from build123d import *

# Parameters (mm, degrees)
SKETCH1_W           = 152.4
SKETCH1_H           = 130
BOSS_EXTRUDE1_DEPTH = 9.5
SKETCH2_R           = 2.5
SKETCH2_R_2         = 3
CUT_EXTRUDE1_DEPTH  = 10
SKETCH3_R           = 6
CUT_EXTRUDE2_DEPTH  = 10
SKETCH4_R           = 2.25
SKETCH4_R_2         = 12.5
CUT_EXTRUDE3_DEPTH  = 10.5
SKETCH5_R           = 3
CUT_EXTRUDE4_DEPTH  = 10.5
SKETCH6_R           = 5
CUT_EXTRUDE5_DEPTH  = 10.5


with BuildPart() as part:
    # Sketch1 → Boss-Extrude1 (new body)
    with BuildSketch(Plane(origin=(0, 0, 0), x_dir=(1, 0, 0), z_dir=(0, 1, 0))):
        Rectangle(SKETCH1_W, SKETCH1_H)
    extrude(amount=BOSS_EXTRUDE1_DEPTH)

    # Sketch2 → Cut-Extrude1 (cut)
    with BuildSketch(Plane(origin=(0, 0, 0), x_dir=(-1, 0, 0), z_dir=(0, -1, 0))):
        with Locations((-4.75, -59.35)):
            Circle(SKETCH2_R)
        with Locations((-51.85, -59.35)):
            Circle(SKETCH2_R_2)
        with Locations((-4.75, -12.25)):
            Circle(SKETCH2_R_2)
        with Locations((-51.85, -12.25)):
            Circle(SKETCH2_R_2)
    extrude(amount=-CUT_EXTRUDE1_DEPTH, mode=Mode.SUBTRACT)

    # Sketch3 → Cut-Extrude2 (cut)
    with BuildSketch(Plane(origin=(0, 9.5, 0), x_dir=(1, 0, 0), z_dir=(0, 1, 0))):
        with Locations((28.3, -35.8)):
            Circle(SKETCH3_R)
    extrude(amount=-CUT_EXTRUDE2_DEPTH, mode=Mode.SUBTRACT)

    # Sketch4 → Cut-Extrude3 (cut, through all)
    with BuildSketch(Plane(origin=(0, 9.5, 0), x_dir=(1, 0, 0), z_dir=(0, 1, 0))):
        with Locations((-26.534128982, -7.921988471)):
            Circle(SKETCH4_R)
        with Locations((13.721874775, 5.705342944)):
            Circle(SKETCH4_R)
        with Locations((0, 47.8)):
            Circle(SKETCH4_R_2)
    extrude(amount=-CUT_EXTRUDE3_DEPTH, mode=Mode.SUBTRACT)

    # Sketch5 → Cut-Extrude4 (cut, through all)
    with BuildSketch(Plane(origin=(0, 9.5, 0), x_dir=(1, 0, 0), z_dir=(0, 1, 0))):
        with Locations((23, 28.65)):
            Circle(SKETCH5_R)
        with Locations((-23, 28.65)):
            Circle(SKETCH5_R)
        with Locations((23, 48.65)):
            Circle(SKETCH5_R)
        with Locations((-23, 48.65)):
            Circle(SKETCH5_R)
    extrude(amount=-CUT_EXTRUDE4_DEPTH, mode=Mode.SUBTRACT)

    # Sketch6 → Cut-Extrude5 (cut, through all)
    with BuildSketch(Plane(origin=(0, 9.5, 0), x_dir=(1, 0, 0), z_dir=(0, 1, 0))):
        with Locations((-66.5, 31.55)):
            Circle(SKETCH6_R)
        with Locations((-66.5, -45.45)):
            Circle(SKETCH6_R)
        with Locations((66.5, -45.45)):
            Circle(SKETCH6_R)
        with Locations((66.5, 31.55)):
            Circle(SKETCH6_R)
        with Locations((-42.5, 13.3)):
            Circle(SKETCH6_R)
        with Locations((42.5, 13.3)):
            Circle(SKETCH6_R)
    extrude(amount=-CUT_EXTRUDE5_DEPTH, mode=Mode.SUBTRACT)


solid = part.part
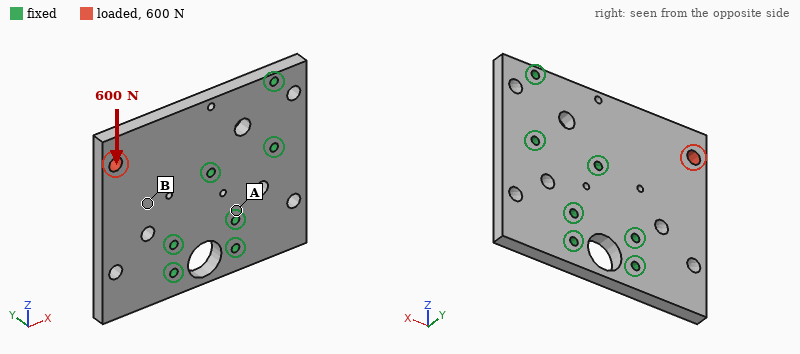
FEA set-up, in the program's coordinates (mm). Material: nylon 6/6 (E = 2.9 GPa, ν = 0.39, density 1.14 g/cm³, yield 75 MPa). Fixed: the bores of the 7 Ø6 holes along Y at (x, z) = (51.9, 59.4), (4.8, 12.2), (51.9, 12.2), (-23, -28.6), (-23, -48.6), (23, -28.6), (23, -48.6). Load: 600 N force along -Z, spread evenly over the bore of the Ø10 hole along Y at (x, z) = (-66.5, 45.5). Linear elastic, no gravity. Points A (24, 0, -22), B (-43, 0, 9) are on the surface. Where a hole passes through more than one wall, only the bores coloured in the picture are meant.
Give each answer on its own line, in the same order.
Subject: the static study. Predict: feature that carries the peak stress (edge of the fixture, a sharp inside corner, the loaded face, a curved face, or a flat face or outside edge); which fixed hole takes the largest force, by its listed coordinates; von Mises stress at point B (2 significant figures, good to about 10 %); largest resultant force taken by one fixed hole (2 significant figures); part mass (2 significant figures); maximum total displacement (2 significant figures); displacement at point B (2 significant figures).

the loaded face
(-23, -28.6)
1.4 MPa
330 N
200 g
0.10 mm
0.030 mm
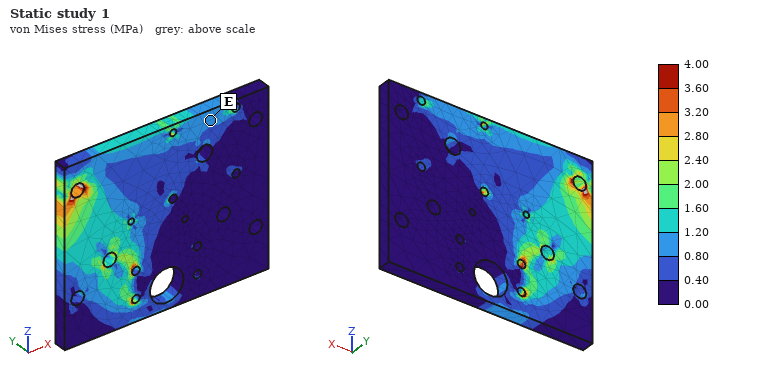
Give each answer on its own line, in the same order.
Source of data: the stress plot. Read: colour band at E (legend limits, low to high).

0.80 to 1.20 MPa
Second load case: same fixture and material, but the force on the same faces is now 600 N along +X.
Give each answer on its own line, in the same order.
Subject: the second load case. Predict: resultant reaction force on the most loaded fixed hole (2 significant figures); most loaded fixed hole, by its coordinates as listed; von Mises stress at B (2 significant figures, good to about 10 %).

300 N
(4.8, 12.2)
0.40 MPa
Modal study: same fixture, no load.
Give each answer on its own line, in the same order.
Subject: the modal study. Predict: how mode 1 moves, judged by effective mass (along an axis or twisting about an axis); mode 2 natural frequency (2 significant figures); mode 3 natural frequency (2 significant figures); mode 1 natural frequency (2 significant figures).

along Y
900 Hz
1200 Hz
430 Hz
